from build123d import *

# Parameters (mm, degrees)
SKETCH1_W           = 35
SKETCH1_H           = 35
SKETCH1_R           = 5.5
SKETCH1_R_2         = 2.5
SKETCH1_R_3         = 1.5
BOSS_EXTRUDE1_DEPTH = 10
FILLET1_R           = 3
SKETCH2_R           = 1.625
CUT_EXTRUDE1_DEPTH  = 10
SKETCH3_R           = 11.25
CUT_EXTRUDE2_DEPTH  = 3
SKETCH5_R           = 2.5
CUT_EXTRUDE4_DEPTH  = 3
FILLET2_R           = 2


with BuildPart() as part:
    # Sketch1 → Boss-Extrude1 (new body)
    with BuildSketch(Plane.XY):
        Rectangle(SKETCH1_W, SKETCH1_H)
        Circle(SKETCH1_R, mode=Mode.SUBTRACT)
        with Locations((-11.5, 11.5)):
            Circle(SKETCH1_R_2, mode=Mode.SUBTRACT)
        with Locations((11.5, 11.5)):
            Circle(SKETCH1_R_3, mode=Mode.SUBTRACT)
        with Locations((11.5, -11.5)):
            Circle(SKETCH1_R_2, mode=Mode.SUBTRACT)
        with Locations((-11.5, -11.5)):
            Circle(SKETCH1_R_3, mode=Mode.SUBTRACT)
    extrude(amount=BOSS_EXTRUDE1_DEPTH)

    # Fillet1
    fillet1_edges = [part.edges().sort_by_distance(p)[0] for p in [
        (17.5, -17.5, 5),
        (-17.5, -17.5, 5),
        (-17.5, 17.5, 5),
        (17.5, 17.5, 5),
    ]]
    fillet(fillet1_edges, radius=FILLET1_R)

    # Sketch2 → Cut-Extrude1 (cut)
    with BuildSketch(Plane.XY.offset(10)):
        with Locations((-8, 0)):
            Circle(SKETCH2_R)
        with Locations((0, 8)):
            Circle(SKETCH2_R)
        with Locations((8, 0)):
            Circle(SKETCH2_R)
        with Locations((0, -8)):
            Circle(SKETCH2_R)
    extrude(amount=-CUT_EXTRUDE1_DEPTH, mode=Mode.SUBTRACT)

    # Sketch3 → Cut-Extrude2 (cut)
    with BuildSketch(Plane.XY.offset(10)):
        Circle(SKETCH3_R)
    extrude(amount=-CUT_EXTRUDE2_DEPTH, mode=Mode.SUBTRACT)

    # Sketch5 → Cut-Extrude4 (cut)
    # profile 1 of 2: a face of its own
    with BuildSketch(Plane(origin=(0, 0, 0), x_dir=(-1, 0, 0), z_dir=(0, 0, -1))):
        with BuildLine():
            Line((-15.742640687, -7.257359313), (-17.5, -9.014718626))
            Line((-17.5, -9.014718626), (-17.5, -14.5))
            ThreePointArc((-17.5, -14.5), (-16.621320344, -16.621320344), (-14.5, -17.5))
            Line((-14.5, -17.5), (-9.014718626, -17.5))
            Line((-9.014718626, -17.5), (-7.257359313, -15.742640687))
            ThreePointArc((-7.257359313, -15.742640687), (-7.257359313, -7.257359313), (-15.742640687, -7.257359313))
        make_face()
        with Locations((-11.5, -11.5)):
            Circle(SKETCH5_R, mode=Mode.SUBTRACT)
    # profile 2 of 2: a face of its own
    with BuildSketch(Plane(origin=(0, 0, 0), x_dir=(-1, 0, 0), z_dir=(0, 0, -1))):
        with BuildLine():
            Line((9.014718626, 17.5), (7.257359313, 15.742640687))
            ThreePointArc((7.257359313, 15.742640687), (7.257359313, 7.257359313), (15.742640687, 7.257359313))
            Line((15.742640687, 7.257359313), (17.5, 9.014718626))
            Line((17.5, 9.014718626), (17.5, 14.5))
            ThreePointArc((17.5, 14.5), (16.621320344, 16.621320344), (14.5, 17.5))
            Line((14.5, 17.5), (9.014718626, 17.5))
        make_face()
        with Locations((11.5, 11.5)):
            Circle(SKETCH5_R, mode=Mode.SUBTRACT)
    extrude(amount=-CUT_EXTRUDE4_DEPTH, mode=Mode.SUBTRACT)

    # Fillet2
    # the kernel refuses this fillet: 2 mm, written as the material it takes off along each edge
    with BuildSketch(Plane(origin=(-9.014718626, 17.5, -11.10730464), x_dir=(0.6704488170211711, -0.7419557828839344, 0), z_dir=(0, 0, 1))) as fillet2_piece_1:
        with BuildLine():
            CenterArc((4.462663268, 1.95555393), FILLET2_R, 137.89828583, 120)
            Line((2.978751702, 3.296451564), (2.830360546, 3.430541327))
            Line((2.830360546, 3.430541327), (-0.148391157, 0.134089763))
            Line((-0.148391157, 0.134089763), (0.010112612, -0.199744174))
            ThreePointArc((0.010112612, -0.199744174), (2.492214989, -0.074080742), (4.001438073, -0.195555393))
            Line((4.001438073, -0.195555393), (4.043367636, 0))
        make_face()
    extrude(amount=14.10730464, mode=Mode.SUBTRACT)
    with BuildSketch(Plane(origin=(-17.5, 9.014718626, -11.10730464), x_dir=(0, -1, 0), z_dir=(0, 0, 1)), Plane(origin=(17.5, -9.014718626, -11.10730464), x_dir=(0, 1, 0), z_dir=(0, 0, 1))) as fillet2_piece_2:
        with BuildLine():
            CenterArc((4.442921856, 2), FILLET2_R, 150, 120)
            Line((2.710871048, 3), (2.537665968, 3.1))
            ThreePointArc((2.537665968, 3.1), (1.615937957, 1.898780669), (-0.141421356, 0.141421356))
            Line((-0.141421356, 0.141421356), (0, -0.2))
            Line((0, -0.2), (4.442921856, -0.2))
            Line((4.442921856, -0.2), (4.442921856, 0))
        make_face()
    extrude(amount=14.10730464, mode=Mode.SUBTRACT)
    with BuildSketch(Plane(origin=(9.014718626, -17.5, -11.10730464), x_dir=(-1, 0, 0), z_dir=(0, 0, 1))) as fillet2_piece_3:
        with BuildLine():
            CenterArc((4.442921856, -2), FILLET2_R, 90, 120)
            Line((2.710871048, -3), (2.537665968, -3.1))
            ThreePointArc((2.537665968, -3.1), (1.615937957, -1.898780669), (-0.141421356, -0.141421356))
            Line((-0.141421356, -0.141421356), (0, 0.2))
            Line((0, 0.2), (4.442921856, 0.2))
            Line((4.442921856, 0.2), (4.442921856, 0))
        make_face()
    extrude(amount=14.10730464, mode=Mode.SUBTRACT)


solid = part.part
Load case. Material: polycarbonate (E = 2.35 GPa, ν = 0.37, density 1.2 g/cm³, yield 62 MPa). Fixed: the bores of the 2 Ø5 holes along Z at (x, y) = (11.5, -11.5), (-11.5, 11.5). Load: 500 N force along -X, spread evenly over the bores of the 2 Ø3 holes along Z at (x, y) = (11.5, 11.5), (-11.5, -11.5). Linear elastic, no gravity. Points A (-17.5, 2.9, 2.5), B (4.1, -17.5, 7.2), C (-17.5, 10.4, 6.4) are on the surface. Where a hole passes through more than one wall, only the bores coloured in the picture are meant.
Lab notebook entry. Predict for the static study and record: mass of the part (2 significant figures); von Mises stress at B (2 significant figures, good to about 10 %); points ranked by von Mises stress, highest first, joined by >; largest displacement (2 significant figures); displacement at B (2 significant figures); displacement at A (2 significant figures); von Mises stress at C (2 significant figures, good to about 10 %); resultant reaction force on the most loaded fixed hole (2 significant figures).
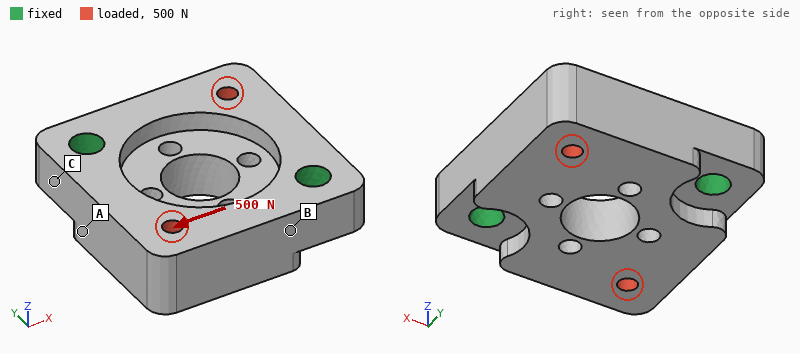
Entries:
11 g
3.0 MPa
B > C > A
38 µm
12 µm
14 µm
1.8 MPa
250 N
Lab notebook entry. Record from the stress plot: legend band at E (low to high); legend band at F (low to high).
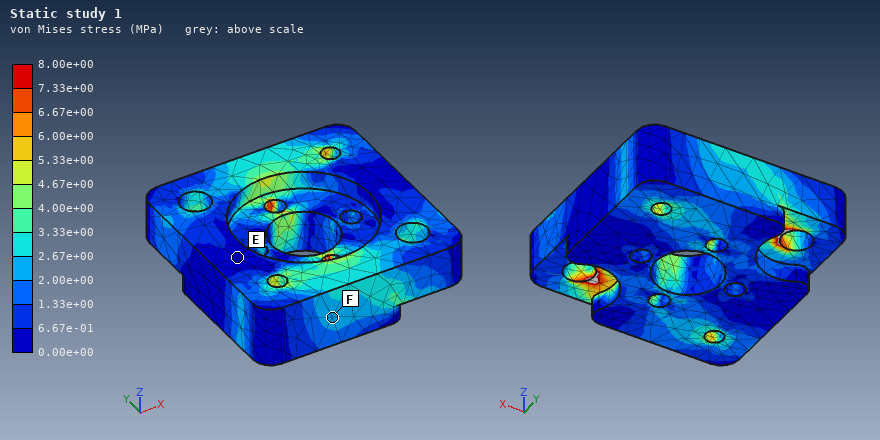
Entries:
0.00e+00 to 6.67e-01 MPa
2.00e+00 to 2.67e+00 MPa
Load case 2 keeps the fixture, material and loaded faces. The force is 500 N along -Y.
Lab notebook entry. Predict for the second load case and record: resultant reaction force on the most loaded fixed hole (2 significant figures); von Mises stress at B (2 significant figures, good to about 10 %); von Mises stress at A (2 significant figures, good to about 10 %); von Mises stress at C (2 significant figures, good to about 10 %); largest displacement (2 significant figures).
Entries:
250 N
0.77 MPa
2.1 MPa
1.6 MPa
38 µm
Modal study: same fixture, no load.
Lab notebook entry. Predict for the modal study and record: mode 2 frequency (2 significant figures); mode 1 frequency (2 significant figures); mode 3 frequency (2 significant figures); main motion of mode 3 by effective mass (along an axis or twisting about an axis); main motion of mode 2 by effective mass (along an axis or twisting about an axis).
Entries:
3600 Hz
2800 Hz
8800 Hz
twisting about Z
along Z
